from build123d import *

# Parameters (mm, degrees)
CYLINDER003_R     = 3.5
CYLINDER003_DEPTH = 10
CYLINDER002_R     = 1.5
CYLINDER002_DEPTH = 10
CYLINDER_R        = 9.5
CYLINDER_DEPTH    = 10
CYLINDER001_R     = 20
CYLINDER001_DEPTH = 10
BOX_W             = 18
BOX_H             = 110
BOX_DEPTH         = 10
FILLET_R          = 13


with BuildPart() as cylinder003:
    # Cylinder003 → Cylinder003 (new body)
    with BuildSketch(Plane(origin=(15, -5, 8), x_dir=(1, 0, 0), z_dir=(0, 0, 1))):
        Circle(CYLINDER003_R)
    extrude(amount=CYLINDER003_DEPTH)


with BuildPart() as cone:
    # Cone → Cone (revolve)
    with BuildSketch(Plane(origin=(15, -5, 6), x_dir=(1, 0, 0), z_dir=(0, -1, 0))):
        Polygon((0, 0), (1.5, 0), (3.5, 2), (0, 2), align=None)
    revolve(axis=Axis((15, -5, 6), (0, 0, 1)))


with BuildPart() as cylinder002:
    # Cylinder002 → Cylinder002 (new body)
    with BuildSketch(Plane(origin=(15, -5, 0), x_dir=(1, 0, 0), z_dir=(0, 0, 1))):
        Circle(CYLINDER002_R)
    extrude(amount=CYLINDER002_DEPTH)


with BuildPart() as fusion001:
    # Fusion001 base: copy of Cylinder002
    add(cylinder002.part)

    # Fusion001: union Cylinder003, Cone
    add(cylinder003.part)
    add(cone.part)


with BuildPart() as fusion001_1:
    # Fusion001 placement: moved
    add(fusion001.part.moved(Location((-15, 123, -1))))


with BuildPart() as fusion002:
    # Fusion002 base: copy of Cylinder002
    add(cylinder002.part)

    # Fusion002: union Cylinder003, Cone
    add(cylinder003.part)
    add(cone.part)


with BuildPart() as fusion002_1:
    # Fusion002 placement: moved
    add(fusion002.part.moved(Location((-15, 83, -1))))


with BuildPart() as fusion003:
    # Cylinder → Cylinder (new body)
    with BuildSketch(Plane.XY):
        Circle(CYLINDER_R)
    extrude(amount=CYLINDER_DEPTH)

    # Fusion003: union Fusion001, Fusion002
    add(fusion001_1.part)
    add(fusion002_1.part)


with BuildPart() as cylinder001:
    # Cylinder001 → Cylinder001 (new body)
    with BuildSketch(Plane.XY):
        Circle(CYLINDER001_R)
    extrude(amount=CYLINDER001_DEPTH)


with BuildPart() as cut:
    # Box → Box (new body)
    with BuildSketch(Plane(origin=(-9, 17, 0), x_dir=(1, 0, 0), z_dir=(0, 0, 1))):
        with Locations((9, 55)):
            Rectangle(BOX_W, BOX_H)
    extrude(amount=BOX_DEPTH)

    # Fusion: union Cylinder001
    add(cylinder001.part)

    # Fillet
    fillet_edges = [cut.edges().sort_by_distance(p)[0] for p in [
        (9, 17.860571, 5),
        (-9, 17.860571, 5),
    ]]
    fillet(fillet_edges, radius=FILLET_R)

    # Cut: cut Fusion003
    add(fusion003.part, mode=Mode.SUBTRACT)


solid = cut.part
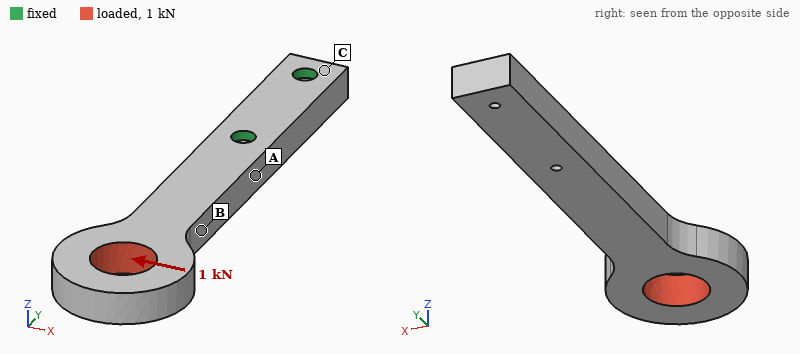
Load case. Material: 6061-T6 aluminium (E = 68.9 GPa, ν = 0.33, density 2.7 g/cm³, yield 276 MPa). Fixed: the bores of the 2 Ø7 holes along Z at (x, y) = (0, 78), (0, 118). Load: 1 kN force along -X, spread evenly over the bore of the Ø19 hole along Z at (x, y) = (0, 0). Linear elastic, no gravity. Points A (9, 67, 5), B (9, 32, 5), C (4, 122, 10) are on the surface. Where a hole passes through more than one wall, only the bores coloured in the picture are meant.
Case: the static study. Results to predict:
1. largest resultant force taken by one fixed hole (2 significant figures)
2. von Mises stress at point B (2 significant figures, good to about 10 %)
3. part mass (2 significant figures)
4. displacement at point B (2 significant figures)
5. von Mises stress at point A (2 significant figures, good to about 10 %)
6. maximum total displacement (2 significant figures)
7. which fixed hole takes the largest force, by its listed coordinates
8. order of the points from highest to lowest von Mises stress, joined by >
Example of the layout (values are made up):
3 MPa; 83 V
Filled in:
2.1 kN; 60 MPa; 78 g; 0.30 mm; 130 MPa; 0.85 mm; (0, 78); A > B > C
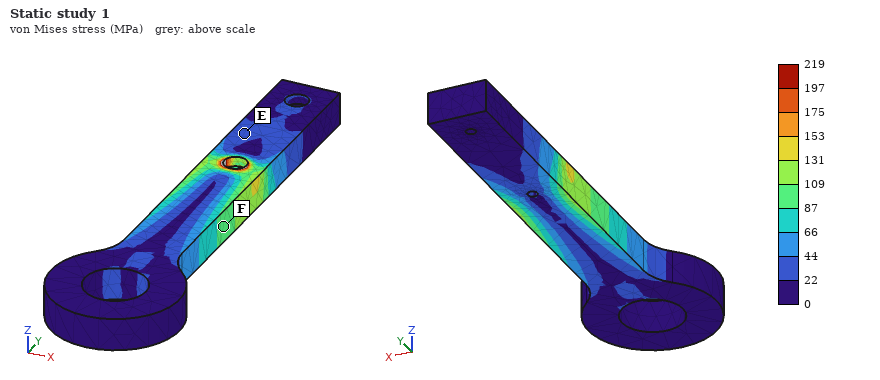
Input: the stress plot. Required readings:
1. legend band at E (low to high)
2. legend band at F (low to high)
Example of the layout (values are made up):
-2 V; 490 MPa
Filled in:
22 to 44 MPa; 87 to 109 MPa
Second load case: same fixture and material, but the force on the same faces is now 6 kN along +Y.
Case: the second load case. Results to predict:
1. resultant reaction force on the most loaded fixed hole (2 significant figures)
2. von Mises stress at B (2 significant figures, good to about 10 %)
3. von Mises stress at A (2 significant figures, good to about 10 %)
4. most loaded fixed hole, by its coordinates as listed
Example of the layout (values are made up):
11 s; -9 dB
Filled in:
4.8 kN; 33 MPa; 30 MPa; (0, 78)
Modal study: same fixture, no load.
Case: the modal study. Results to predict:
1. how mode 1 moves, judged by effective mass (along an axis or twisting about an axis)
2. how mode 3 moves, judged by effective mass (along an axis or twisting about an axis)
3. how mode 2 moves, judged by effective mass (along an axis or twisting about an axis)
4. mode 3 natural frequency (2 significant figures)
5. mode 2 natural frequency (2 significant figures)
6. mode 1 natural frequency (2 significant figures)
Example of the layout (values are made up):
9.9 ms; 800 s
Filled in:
along Z; twisting about Y; along X; 3000 Hz; 1100 Hz; 690 Hz
